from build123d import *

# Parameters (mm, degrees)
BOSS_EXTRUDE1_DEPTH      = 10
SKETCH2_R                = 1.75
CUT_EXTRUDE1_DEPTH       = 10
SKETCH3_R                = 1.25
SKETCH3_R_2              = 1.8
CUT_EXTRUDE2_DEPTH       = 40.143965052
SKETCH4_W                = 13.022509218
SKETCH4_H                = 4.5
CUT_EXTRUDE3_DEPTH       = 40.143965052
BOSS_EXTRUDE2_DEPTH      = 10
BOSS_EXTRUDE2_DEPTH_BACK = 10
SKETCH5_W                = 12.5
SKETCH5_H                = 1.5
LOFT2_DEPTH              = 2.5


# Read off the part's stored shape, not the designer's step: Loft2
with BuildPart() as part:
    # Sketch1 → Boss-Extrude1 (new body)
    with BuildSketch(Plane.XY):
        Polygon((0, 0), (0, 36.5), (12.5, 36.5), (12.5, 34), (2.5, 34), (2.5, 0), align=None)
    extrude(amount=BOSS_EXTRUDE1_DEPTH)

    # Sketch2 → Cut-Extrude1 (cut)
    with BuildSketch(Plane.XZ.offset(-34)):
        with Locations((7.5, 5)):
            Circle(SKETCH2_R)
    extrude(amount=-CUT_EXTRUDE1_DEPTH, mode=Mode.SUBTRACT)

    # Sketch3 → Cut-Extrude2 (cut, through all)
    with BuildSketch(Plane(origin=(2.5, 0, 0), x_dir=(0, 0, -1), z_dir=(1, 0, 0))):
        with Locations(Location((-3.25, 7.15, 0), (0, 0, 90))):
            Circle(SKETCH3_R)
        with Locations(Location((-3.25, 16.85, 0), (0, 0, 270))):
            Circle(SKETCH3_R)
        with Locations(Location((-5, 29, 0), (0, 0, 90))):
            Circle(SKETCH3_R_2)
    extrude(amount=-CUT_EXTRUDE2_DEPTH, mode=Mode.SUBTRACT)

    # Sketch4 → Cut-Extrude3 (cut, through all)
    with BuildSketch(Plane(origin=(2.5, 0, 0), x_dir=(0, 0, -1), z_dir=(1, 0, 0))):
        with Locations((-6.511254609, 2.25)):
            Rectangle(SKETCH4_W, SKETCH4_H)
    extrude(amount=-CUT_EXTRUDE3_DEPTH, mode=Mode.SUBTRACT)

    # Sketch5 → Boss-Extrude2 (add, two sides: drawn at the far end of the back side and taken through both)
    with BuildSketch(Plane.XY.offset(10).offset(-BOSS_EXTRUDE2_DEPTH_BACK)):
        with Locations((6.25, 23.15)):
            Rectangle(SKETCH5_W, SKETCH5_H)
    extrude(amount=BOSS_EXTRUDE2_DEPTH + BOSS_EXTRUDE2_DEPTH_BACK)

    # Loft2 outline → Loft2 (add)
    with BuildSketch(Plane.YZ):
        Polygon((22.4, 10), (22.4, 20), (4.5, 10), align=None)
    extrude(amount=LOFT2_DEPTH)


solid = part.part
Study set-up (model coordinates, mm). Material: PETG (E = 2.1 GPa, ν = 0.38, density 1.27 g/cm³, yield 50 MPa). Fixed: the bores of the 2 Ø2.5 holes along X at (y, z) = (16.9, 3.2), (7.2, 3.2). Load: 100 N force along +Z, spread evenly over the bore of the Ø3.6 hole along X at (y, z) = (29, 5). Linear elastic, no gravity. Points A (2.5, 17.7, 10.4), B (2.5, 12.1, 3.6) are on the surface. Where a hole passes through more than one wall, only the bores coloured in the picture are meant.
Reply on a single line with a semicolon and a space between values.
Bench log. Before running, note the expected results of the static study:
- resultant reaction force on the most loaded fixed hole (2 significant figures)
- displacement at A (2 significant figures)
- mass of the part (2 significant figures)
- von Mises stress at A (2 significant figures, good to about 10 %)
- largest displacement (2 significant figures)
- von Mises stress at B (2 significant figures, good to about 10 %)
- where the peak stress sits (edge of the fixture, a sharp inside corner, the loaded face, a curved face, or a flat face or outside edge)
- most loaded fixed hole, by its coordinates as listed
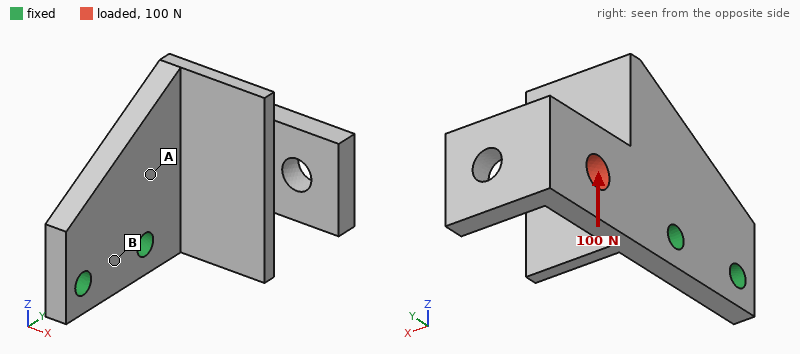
190 N; 0.065 mm; 2.0 g; 8.5 MPa; 0.39 mm; 3.0 MPa; edge of the fixture; (16.9, 3.2)
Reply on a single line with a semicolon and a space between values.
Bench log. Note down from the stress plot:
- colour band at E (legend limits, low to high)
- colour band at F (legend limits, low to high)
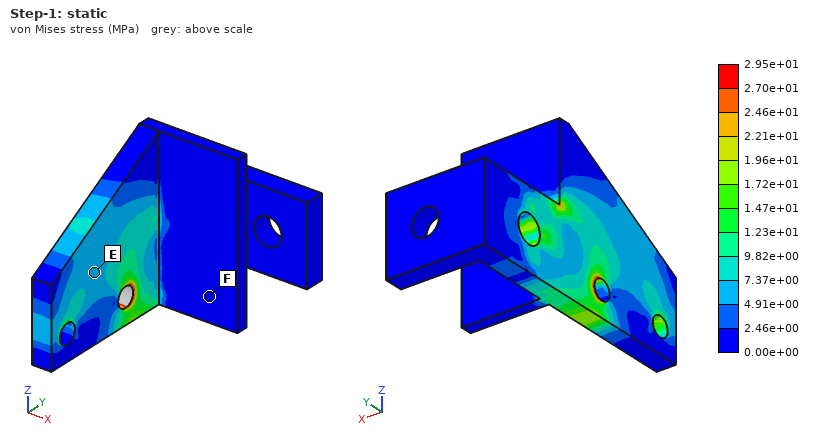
4.91e+00 to 7.37e+00 MPa; 0.00e+00 to 2.46e+00 MPa
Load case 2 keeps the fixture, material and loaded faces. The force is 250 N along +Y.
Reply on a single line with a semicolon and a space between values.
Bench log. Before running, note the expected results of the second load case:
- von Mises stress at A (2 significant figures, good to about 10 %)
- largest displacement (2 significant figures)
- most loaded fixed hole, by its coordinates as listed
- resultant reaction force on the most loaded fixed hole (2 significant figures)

3.7 MPa; 91 µm; (16.9, 3.2); 210 N
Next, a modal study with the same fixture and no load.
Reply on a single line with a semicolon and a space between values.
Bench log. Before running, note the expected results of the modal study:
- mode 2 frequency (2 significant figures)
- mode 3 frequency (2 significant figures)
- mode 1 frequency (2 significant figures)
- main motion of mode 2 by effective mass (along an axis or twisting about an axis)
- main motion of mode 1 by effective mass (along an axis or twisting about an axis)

1400 Hz; 2100 Hz; 810 Hz; along Z; along X
